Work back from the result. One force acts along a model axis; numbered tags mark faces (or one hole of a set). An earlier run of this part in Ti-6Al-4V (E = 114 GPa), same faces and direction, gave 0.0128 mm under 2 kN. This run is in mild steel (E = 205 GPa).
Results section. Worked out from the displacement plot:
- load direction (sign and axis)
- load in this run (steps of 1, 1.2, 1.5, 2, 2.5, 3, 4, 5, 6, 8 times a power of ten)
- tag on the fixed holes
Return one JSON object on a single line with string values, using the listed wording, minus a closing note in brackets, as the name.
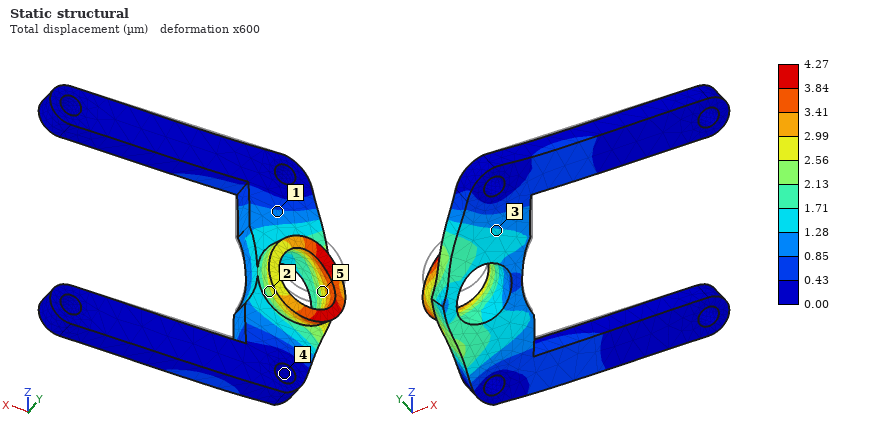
{"load direction": "-Z", "load in this run": "1.2 kN", "tag on the fixed holes": "4"}
